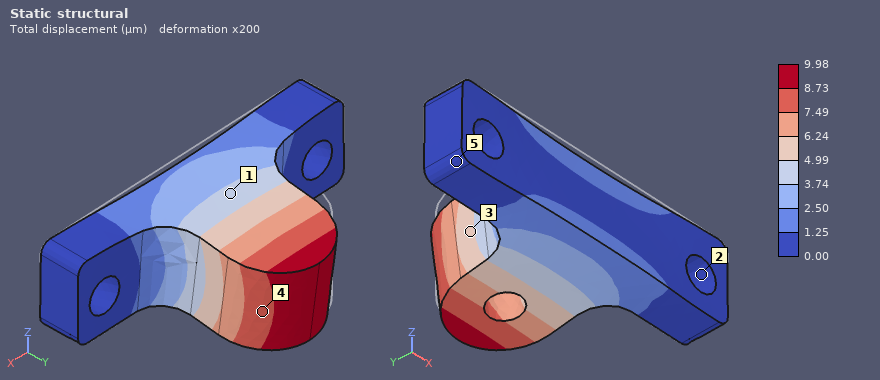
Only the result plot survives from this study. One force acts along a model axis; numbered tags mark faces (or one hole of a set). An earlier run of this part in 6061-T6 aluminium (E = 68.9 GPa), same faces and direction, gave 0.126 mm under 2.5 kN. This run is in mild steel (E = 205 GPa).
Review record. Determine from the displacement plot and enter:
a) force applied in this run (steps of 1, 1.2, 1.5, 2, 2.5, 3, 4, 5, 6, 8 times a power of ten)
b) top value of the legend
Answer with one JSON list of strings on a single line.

["600 N", "9.98 µm"]
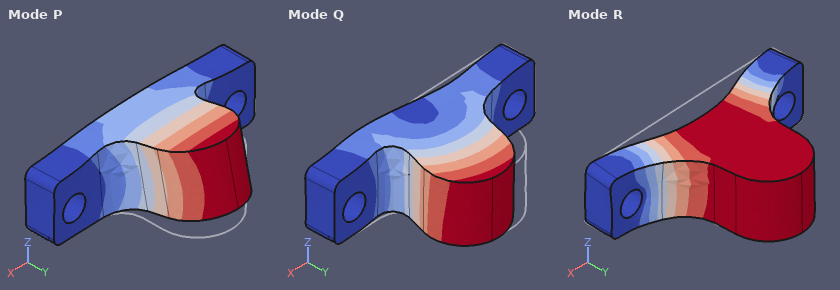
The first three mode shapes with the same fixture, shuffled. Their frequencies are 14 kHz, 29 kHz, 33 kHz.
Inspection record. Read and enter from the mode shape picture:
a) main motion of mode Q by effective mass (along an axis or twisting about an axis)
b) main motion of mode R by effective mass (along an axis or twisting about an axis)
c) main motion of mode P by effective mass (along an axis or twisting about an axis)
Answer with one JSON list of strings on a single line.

["along X", "along Y", "along Z"]
